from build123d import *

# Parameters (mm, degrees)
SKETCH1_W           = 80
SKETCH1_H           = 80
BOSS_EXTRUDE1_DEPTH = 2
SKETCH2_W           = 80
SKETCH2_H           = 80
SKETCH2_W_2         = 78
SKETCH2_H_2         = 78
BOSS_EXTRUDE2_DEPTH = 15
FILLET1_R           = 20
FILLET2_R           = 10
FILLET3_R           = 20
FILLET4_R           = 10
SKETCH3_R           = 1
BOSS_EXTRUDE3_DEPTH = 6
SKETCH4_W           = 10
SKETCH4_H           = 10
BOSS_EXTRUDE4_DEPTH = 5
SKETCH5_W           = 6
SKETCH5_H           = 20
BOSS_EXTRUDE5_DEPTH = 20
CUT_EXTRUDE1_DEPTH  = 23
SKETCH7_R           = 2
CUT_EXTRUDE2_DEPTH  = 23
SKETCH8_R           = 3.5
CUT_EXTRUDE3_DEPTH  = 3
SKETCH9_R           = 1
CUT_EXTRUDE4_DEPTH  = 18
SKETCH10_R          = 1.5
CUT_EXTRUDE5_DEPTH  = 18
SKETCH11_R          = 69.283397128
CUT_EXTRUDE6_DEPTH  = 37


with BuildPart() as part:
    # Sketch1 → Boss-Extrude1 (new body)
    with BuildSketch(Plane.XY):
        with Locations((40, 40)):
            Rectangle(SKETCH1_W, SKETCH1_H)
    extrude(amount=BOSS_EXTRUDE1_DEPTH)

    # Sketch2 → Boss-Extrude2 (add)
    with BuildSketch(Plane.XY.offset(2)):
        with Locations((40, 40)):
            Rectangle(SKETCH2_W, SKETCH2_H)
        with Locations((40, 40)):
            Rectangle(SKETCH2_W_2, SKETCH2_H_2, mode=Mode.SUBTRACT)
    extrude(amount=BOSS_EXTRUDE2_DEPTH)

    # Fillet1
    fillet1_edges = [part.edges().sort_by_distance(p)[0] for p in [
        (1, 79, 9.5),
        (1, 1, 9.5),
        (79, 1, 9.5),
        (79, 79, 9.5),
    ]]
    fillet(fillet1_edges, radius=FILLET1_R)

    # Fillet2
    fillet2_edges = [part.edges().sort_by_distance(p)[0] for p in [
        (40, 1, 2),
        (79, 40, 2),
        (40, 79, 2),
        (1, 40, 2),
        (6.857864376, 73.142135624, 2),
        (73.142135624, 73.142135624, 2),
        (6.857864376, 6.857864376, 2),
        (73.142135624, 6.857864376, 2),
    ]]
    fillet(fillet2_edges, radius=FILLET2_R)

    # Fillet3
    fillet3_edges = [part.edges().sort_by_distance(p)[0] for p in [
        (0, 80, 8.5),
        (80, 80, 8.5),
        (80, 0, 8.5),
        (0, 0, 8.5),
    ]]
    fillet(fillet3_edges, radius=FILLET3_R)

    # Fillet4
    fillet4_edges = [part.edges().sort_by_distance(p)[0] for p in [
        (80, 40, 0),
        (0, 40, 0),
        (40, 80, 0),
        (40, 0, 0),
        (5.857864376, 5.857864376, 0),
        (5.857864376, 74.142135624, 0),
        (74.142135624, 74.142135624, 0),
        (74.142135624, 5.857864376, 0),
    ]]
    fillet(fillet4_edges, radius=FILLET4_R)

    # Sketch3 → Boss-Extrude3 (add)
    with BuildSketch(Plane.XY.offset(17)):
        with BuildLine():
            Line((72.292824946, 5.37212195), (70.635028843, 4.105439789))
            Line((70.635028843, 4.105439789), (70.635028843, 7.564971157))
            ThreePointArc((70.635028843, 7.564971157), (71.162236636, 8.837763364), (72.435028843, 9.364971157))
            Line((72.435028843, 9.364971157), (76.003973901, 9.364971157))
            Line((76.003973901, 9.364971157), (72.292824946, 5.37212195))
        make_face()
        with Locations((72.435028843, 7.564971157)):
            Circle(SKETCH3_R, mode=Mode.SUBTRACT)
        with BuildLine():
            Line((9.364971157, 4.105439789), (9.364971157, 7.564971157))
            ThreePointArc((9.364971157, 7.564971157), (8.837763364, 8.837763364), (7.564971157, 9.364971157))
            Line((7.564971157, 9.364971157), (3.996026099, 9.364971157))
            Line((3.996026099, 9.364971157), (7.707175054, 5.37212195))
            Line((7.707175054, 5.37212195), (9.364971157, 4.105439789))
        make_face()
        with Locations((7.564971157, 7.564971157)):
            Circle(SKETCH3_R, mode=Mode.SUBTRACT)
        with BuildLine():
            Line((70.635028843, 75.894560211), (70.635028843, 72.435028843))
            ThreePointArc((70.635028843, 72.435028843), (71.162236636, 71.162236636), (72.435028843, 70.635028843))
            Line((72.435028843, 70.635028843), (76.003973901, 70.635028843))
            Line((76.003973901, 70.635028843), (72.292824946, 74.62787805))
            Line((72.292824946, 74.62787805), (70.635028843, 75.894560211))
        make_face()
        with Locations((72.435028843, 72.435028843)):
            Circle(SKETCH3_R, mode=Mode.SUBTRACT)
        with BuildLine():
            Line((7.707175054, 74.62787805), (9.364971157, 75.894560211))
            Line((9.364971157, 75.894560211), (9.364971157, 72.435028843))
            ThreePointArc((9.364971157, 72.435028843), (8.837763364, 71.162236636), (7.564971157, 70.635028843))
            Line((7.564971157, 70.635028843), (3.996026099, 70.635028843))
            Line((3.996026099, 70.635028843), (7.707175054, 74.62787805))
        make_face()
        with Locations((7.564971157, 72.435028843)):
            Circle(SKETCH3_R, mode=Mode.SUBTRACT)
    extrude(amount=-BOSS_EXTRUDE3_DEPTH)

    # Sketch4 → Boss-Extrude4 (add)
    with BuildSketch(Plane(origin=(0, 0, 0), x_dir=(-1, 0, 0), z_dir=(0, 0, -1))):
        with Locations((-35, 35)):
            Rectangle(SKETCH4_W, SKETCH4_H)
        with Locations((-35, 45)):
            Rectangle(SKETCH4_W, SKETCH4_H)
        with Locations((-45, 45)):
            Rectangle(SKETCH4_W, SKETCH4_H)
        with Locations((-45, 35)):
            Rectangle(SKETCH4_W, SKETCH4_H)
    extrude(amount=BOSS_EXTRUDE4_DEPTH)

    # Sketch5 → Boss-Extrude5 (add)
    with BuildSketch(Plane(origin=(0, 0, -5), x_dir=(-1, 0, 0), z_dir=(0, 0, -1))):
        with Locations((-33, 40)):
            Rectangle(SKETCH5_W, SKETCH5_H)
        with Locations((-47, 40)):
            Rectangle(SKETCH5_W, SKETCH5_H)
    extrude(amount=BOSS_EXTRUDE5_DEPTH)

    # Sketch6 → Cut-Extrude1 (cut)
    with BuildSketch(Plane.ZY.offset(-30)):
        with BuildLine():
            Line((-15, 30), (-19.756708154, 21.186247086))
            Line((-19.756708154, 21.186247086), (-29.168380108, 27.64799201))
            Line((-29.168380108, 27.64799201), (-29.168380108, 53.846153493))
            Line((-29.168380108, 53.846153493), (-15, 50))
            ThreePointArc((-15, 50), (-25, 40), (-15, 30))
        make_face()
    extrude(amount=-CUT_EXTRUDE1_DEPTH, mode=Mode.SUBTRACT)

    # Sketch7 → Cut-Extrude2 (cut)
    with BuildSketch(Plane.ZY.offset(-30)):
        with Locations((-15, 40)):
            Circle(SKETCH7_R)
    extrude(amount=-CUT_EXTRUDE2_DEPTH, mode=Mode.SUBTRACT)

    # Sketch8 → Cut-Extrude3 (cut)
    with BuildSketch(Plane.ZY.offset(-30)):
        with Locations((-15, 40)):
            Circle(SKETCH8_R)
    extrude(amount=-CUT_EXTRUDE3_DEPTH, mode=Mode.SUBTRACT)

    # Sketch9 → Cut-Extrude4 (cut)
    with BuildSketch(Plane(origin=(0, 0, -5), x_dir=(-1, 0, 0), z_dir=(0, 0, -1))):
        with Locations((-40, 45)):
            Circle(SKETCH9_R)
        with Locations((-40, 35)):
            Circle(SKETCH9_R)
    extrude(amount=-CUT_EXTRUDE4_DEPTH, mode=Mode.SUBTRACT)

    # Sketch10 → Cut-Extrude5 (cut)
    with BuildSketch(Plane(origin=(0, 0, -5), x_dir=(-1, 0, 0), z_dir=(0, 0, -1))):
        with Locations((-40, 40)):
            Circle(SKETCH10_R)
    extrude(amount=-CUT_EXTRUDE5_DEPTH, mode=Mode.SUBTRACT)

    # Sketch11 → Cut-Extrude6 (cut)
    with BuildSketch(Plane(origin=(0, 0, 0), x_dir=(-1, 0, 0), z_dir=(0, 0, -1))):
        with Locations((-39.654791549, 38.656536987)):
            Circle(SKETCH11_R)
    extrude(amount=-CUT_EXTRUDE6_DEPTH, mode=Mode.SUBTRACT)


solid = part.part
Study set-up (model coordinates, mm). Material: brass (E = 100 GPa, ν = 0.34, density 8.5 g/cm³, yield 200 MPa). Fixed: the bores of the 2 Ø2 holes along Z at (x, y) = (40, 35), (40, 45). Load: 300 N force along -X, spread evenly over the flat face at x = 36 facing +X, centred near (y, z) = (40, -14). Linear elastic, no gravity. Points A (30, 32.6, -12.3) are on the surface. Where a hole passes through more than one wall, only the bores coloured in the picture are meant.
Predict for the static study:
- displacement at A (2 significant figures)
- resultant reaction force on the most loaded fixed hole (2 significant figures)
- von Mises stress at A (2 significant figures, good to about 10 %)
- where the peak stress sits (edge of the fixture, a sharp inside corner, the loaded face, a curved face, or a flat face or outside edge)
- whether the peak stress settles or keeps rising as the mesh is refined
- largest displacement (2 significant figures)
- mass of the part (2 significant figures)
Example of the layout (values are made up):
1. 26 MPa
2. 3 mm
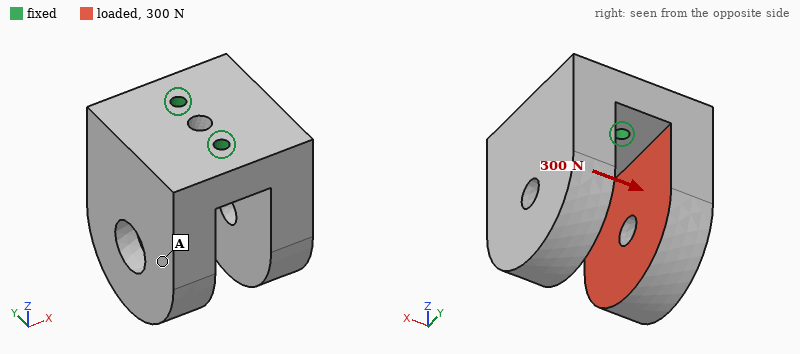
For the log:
1. 17 µm
2. 150 N
3. 10 MPa
4. edge of the fixture
5. keeps rising
6. 37 µm
7. 51 g
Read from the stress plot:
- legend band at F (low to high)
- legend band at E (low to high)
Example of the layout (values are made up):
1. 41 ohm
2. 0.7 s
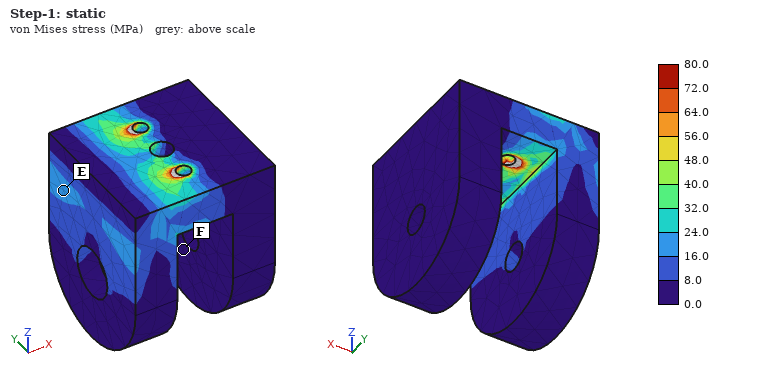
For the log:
1. 0.0 to 8.0 MPa
2. 16.0 to 24.0 MPa
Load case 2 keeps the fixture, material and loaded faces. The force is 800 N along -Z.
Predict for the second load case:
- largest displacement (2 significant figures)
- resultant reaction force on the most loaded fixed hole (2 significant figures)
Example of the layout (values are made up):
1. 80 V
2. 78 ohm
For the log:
1. 5.9 µm
2. 400 N
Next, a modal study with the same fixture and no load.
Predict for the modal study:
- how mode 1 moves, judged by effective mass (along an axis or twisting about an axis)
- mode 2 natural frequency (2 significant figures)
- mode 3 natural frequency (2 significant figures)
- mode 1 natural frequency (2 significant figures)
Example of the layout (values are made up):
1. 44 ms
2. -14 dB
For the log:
1. along X
2. 4500 Hz
3. 7700 Hz
4. 4000 Hz
